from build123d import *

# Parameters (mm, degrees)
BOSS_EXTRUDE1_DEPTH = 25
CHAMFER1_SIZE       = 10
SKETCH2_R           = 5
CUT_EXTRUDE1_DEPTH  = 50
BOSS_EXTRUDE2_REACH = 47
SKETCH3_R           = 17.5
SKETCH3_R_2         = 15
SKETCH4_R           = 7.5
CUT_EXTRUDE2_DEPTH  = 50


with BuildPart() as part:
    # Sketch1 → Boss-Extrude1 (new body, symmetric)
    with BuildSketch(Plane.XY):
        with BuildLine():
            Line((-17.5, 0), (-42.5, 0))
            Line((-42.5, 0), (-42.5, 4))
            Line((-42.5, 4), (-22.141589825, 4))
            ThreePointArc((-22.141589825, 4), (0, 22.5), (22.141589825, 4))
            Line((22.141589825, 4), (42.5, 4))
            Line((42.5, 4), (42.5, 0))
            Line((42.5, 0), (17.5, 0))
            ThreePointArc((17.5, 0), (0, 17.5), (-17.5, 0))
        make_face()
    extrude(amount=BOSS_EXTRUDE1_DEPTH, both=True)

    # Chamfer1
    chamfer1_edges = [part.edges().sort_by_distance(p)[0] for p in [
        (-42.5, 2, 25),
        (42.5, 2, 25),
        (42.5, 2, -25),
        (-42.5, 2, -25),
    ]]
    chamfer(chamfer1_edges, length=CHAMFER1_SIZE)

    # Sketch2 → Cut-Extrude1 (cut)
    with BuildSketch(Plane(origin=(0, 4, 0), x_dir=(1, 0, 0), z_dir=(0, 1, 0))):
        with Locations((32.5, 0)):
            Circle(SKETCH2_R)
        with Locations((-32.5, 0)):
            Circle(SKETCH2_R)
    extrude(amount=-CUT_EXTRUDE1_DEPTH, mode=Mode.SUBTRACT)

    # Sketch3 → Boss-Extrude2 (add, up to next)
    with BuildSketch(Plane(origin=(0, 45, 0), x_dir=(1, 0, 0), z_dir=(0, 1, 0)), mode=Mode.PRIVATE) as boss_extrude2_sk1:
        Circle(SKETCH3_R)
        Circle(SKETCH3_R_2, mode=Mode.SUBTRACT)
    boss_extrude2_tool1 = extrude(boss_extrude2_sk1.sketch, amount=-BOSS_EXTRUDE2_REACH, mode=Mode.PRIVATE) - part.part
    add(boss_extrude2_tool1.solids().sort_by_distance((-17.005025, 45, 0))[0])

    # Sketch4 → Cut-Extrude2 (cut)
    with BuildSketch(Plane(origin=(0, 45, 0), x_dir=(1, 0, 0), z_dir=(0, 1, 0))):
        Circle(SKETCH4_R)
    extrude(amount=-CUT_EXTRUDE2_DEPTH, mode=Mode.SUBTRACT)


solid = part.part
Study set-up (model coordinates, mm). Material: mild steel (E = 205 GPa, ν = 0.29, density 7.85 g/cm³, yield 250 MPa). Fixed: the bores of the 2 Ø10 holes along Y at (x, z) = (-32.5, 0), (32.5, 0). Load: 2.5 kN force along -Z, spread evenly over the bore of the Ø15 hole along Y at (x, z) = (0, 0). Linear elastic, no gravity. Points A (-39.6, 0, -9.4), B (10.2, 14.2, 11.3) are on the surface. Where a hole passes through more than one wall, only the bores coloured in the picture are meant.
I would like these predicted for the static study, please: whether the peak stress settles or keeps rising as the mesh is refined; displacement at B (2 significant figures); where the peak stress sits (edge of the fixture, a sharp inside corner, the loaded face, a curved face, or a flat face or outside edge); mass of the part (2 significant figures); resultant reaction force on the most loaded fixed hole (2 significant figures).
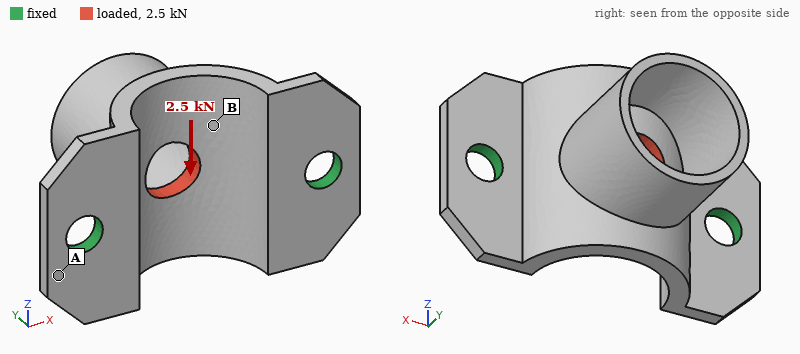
keeps rising
36 µm
edge of the fixture
220 g
1.3 kN
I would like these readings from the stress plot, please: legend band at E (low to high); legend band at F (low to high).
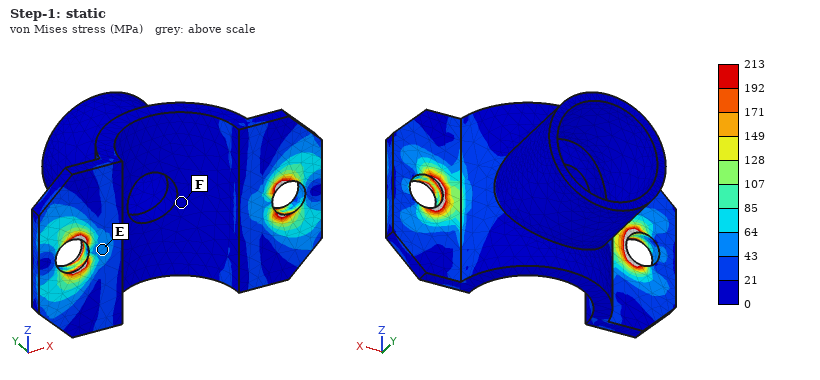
43 to 64 MPa
0 to 21 MPa
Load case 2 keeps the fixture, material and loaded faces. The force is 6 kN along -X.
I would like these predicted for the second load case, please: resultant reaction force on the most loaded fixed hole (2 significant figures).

3.5 kN
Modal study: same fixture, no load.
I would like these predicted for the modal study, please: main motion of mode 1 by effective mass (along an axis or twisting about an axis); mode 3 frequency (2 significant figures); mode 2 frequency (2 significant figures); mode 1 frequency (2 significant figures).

along Z
7500 Hz
7400 Hz
2300 Hz
